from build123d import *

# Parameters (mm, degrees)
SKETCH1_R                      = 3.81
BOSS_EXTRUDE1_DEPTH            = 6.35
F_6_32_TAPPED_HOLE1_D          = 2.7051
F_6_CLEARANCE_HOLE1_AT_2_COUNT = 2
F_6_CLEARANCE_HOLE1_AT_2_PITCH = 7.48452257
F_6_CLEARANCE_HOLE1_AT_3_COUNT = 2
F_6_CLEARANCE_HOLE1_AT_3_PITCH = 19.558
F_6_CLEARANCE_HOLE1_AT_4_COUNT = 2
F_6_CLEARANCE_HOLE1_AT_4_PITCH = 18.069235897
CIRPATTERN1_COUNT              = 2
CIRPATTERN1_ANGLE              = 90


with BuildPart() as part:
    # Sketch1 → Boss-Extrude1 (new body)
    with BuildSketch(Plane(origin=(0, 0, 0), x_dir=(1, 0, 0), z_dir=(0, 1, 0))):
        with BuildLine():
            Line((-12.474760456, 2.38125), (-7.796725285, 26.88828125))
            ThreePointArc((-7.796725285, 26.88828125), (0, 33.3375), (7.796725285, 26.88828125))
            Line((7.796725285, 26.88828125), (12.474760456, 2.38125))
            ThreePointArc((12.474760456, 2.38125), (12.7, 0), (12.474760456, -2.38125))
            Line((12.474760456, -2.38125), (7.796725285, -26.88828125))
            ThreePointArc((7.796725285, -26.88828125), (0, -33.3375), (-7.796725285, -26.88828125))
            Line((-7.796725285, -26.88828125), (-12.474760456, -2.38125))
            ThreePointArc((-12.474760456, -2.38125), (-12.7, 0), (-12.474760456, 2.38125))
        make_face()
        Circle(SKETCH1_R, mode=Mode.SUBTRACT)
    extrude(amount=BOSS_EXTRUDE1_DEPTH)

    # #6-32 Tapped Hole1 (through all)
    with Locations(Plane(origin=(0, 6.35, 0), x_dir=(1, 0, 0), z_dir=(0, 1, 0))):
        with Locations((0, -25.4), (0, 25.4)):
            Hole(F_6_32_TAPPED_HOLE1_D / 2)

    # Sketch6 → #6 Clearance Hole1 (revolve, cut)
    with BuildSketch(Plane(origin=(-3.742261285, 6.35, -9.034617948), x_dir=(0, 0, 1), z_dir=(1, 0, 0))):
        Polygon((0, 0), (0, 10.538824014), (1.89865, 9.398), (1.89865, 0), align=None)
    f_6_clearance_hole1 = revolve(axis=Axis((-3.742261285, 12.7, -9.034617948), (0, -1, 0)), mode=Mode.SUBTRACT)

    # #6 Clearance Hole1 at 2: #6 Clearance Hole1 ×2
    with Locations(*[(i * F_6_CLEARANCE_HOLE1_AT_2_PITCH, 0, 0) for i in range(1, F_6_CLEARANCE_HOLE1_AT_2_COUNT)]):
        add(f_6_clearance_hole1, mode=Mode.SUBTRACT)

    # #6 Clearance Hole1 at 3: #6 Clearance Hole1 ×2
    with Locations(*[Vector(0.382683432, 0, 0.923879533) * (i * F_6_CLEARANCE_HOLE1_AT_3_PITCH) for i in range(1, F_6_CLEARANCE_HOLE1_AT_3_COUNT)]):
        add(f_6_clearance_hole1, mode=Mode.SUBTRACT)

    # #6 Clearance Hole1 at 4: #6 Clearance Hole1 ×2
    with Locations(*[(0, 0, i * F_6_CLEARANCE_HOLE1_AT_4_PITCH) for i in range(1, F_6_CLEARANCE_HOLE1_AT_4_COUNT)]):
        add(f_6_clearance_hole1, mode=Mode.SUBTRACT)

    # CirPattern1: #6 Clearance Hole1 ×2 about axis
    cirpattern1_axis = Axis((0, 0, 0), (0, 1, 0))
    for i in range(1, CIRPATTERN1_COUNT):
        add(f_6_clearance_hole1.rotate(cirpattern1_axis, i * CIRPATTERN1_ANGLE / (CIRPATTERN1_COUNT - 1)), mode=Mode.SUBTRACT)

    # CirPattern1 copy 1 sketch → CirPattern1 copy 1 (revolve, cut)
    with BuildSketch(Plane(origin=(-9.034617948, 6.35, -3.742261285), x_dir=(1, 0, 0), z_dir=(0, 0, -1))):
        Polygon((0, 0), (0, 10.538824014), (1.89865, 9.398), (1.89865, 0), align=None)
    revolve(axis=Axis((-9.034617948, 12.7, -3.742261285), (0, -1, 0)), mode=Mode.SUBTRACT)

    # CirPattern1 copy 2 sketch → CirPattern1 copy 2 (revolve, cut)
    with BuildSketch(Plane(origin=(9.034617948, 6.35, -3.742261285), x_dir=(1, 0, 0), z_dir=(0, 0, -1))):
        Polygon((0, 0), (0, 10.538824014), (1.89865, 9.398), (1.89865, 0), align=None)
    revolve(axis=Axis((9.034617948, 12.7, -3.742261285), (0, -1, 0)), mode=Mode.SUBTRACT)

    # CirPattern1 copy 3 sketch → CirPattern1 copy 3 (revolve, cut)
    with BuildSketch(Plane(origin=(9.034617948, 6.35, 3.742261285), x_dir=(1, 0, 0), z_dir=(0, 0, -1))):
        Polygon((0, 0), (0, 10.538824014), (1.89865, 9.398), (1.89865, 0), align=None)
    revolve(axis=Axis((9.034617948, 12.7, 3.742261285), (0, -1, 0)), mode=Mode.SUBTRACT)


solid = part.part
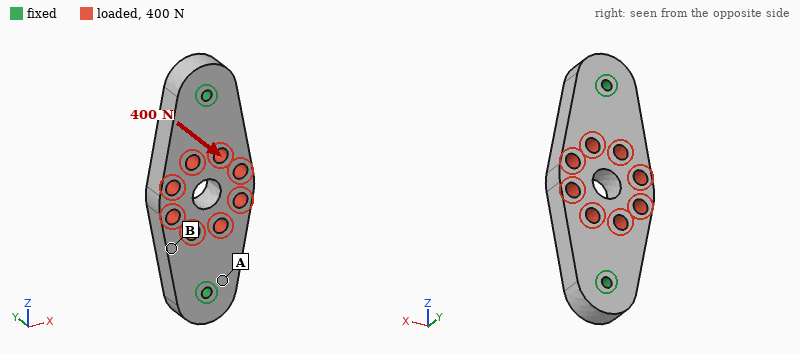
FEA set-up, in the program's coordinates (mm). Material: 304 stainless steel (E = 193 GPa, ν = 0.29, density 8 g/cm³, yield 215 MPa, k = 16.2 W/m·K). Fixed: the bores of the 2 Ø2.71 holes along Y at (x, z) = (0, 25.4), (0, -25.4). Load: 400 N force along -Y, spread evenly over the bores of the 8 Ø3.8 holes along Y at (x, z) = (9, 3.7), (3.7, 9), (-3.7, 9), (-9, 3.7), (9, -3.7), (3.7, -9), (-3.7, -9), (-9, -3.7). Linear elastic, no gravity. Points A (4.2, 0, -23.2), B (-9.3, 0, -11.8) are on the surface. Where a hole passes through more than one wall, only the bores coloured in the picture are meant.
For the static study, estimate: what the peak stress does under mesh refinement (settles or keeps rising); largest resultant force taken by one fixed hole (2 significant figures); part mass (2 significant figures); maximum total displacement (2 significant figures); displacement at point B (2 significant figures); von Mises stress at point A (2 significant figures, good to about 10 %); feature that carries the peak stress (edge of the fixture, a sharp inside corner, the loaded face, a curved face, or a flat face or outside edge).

keeps rising
200 N
57 g
5.6 µm
3.4 µm
12 MPa
edge of the fixture
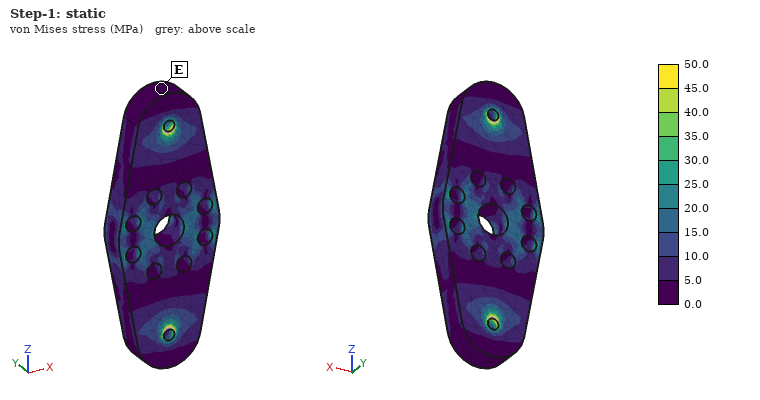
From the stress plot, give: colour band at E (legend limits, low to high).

0.0 to 5.0 MPa
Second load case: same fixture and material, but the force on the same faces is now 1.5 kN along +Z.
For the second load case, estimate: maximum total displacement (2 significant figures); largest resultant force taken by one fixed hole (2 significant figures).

1.0 µm
750 N
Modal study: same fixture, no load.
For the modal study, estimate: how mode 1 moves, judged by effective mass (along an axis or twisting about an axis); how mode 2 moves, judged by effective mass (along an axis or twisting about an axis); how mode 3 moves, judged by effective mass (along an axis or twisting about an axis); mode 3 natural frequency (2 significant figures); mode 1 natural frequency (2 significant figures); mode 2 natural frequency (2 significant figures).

along Y
twisting about Z
along X
16 kHz
9300 Hz
13 kHz
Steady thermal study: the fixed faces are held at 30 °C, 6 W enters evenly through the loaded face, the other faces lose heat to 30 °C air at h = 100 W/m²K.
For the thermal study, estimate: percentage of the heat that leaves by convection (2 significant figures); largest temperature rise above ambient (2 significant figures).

55 %
20 K
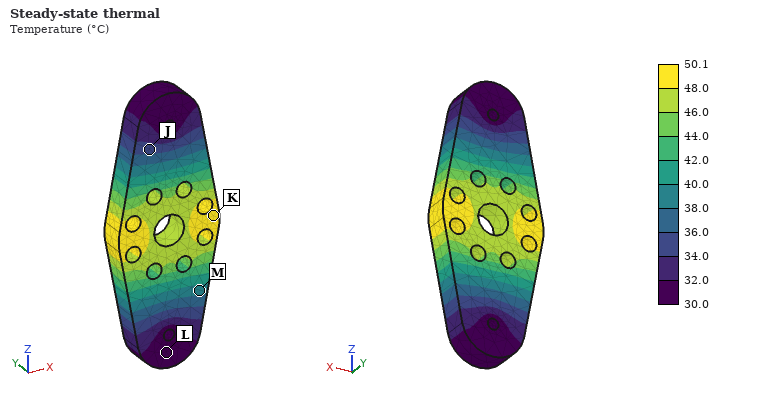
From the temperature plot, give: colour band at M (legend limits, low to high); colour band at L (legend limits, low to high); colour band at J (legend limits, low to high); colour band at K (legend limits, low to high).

38.0 to 40.0 °C
30.0 to 32.0 °C
34.0 to 36.0 °C
48.0 to 50.1 °C
